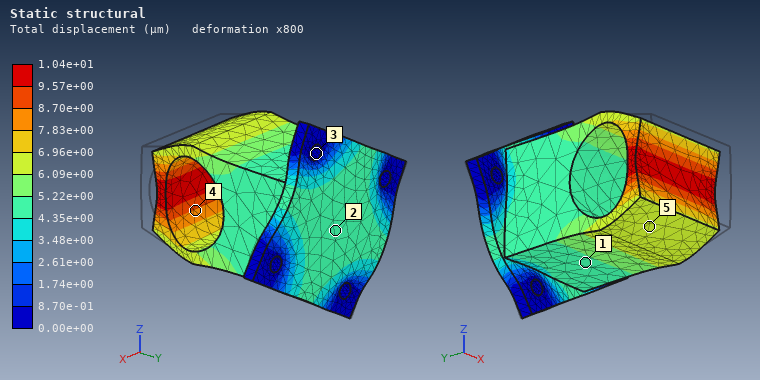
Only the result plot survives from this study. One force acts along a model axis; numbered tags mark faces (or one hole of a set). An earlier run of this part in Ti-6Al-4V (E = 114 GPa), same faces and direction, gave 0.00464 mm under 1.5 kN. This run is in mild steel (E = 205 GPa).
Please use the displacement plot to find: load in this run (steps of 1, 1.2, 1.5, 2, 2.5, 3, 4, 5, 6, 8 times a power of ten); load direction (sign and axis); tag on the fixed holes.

6 kN
+Y
3
